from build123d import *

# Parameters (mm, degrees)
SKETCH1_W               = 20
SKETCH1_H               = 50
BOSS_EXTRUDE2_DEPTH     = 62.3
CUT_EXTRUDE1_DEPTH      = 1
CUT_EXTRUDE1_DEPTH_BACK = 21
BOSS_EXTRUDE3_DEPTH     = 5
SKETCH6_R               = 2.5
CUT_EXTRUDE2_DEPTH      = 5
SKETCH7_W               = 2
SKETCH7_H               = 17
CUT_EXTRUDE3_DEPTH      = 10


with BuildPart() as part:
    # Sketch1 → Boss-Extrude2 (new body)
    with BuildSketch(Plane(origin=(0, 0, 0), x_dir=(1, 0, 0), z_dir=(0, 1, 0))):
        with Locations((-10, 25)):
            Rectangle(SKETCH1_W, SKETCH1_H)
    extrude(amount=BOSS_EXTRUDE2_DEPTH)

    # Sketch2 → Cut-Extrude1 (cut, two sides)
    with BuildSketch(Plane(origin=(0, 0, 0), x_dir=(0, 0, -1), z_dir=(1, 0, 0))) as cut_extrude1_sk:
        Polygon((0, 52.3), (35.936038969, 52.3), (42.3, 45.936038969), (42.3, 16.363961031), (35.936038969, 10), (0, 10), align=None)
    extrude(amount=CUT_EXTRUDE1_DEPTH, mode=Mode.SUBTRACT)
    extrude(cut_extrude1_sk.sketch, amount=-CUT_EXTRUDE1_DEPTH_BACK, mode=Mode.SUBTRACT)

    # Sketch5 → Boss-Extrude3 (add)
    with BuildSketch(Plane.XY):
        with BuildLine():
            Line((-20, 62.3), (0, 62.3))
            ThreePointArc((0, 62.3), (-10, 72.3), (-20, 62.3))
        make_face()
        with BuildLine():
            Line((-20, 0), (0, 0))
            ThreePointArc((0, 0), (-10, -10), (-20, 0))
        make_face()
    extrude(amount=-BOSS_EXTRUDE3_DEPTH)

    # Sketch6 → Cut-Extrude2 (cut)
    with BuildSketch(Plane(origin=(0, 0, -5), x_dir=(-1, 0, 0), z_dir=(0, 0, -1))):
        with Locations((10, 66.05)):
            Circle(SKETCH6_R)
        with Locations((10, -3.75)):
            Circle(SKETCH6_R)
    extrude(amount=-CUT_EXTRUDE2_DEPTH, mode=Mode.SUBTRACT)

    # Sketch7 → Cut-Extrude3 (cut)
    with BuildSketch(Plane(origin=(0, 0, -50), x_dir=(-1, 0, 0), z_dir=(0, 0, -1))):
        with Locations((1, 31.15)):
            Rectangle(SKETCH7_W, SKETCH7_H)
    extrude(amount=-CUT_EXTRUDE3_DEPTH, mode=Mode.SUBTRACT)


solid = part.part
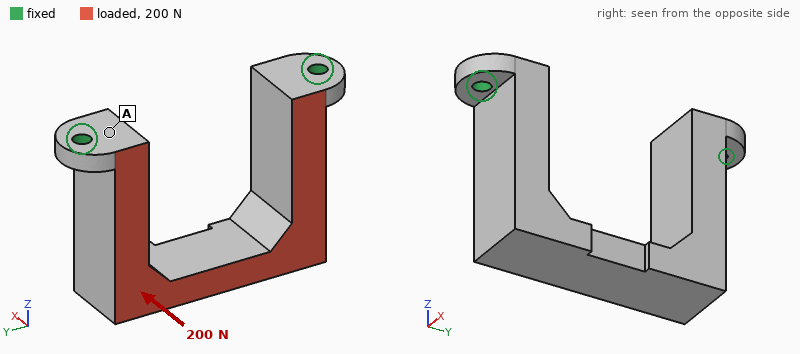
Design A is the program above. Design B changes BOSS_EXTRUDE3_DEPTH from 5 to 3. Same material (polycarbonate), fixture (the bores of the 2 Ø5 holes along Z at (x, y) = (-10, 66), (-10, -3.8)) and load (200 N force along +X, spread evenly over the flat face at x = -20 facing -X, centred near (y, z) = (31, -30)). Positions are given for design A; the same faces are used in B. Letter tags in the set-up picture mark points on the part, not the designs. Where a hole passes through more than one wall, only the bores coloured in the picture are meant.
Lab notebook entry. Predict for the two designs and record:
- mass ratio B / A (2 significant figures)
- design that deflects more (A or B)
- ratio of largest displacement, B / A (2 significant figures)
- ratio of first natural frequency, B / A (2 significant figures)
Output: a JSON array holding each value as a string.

["0.98", "B", "2.6", "0.62"]
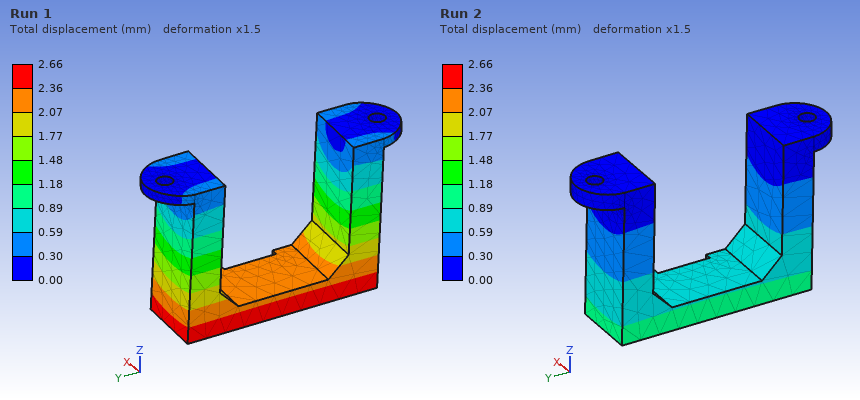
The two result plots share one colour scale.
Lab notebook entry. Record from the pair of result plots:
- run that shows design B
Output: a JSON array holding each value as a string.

["Run 1"]
